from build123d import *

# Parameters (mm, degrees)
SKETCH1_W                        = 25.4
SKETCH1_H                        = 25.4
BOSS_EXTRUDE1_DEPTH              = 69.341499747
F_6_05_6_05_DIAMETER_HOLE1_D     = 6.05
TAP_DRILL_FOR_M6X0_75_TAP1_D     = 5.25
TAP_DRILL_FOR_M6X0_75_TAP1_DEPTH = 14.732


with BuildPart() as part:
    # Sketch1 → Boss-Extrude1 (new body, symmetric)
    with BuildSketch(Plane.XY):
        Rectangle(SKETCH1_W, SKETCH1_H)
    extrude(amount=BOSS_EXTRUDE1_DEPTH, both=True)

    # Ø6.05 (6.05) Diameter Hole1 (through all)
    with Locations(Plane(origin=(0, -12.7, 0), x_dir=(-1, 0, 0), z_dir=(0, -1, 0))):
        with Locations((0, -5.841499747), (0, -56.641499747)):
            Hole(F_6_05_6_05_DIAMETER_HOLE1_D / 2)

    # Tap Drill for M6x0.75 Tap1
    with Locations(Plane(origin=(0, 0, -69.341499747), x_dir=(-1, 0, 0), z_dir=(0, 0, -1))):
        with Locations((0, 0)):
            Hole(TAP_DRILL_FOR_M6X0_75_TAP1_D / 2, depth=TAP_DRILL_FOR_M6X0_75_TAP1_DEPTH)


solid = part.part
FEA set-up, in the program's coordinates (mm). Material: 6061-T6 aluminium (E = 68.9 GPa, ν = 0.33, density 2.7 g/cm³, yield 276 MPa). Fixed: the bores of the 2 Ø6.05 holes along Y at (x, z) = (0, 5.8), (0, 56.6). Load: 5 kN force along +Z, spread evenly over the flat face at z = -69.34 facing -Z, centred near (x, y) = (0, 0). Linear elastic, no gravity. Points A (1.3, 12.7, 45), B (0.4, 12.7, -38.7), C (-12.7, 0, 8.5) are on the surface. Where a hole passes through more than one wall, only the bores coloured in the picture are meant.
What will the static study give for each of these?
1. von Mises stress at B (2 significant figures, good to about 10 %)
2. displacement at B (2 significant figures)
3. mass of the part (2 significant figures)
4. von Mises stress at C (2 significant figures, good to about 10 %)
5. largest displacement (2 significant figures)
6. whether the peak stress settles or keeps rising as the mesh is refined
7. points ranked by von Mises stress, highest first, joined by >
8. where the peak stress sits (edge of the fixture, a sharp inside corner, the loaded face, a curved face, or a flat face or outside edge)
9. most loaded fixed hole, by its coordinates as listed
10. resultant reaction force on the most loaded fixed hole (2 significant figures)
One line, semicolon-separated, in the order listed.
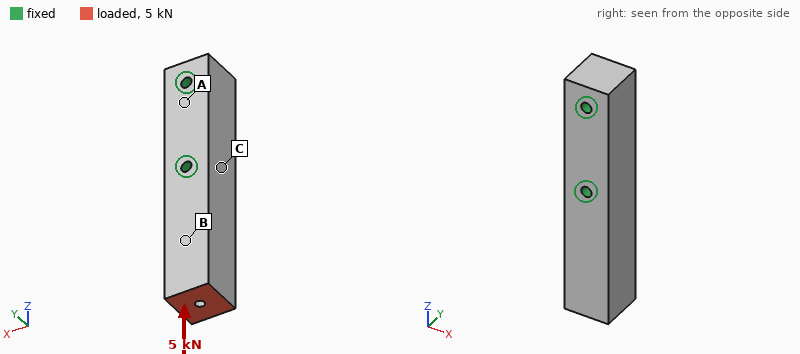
7.7 MPa; 5.4 µm; 240 g; 4.0 MPa; 8.9 µm; keeps rising; B > C > A; edge of the fixture; (0, 5.8); 4.6 kN
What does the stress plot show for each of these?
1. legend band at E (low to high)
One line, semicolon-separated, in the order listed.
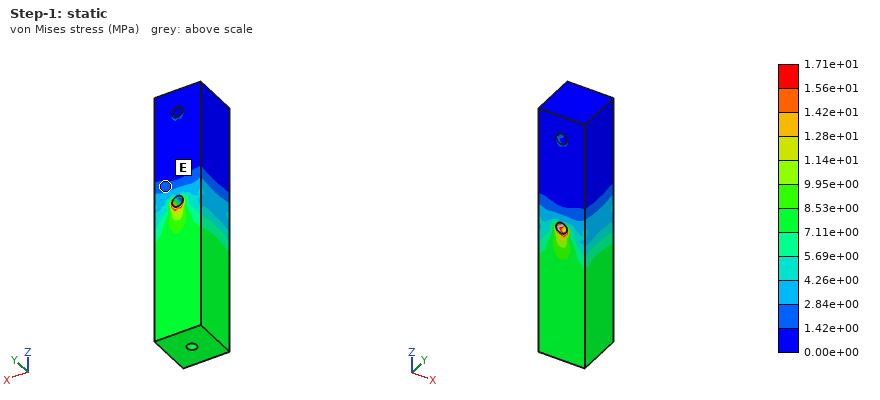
1.42e+00 to 2.84e+00 MPa
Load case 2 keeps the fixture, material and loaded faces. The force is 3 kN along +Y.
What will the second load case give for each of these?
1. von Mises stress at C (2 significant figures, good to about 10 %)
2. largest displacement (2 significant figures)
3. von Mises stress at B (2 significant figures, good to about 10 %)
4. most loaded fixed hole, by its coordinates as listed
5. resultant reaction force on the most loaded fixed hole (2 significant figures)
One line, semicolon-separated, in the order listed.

16 MPa; 0.21 mm; 34 MPa; (0, 5.8); 3.9 kN
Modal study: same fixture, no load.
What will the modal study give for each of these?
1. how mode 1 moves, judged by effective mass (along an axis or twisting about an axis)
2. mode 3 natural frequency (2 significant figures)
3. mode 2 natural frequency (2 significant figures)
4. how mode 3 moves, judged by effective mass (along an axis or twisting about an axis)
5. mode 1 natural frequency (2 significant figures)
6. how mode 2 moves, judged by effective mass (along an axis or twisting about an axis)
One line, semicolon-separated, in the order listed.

along X; 9300 Hz; 3300 Hz; twisting about Z; 2800 Hz; along Y
